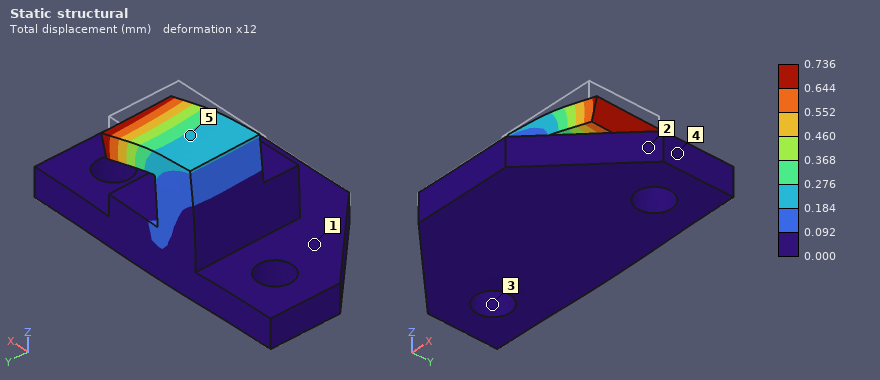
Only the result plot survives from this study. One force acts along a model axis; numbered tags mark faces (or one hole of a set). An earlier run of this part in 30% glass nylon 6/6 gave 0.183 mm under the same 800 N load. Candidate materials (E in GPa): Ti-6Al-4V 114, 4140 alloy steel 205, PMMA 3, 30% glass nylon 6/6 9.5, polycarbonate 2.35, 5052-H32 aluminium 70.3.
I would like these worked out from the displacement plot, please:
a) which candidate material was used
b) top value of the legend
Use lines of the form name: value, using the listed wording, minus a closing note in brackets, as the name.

which candidate material was used: polycarbonate
top value of the legend: 0.736 mm
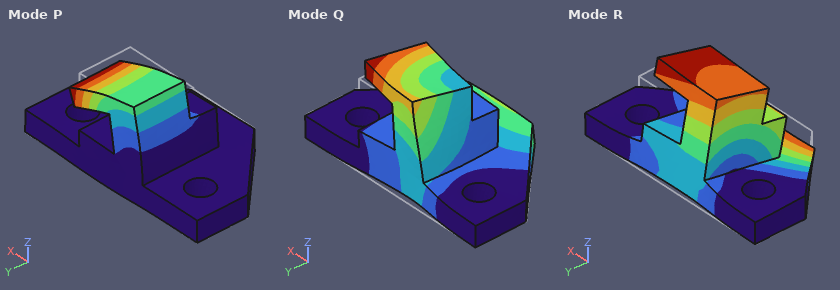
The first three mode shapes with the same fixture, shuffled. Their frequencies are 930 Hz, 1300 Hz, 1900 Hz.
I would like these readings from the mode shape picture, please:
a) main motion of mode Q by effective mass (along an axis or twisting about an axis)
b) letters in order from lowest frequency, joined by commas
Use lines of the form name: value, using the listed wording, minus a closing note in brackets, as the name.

main motion of mode Q by effective mass: along Z
letters in order from lowest frequency, joined by commas: R, P, Q
